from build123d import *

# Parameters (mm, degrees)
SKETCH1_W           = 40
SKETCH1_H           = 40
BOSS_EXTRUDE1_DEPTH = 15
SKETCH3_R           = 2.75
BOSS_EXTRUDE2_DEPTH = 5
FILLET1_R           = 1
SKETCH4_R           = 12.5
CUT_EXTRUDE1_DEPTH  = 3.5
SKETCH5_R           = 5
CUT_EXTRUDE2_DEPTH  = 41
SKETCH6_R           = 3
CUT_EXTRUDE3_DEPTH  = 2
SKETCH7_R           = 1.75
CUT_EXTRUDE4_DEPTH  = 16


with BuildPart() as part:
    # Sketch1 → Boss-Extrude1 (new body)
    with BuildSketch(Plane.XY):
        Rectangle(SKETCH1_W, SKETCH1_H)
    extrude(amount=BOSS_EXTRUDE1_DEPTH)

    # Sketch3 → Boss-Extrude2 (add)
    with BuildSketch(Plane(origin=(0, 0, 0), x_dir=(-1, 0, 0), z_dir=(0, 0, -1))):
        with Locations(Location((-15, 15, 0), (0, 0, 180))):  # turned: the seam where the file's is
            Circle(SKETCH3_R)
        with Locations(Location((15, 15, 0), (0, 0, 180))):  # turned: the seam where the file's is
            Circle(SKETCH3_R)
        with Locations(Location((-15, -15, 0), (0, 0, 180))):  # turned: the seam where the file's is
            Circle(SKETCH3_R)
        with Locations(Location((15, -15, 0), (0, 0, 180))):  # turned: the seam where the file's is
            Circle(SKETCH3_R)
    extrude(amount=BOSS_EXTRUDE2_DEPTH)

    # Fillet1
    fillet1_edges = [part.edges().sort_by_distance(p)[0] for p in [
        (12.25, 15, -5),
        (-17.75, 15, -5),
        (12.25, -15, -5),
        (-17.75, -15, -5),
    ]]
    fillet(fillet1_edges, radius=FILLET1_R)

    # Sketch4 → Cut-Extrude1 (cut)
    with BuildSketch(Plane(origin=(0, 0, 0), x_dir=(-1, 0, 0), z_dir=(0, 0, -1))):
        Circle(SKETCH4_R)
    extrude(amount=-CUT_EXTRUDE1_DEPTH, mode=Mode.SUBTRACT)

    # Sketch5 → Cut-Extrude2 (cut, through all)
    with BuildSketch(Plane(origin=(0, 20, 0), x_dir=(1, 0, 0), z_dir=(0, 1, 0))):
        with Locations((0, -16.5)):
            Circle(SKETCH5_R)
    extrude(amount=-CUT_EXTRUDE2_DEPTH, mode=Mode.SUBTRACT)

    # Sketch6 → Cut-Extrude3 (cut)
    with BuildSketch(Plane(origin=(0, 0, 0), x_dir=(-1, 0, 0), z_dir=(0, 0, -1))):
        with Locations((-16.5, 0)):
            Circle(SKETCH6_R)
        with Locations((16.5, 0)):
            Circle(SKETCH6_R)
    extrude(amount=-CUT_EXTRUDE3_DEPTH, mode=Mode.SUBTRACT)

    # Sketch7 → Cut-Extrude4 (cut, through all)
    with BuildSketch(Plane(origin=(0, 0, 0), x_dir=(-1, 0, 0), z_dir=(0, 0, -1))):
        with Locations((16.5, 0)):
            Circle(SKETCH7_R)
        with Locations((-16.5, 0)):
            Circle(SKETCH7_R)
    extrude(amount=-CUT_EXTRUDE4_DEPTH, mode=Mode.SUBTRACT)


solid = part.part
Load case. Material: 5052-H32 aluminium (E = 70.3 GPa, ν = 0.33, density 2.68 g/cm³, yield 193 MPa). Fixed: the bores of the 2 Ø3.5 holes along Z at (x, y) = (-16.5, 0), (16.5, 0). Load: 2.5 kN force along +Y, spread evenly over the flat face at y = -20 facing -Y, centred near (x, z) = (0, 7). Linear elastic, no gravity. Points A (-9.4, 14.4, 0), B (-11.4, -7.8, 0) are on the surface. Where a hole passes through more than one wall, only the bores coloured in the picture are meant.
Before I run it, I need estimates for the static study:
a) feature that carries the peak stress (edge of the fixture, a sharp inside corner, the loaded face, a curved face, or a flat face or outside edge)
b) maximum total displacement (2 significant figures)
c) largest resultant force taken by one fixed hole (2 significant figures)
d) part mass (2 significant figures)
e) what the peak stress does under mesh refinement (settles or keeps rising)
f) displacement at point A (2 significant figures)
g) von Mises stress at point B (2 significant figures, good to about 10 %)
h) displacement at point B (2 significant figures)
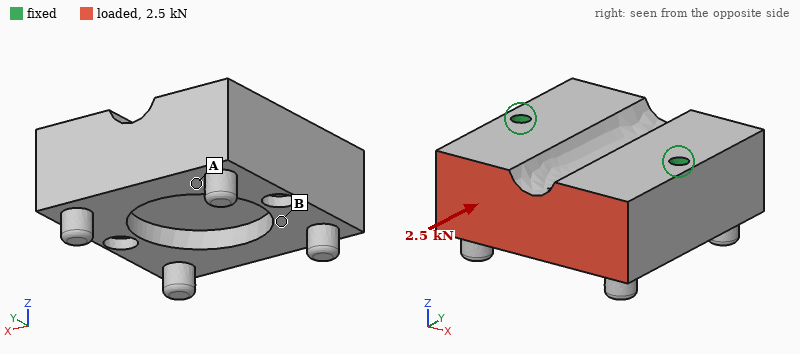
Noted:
edge of the fixture
3.7 µm
1.3 kN
57 g
keeps rising
0.77 µm
7.1 MPa
1.7 µm
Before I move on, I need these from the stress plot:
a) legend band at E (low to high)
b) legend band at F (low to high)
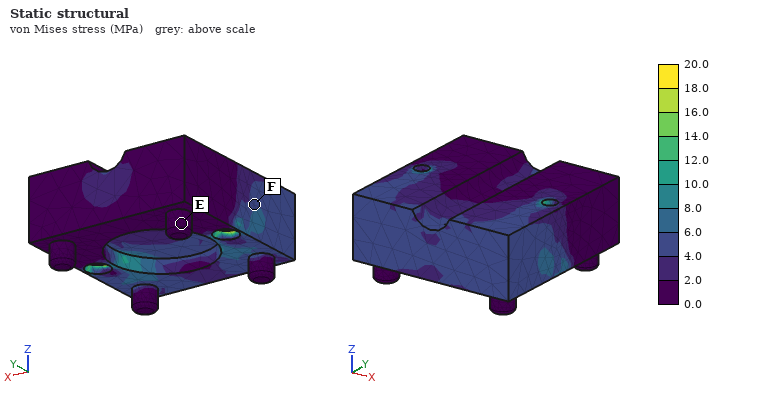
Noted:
0.0 to 2.0 MPa
4.0 to 6.0 MPa
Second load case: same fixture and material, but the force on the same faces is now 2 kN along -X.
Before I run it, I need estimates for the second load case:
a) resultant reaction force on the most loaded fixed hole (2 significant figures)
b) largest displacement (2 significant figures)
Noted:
1.5 kN
6.4 µm
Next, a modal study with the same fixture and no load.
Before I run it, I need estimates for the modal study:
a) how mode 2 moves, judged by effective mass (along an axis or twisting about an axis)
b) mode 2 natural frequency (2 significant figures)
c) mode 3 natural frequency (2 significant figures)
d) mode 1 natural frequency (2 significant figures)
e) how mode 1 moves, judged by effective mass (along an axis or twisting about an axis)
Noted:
along Z
17 kHz
23 kHz
14 kHz
twisting about X
